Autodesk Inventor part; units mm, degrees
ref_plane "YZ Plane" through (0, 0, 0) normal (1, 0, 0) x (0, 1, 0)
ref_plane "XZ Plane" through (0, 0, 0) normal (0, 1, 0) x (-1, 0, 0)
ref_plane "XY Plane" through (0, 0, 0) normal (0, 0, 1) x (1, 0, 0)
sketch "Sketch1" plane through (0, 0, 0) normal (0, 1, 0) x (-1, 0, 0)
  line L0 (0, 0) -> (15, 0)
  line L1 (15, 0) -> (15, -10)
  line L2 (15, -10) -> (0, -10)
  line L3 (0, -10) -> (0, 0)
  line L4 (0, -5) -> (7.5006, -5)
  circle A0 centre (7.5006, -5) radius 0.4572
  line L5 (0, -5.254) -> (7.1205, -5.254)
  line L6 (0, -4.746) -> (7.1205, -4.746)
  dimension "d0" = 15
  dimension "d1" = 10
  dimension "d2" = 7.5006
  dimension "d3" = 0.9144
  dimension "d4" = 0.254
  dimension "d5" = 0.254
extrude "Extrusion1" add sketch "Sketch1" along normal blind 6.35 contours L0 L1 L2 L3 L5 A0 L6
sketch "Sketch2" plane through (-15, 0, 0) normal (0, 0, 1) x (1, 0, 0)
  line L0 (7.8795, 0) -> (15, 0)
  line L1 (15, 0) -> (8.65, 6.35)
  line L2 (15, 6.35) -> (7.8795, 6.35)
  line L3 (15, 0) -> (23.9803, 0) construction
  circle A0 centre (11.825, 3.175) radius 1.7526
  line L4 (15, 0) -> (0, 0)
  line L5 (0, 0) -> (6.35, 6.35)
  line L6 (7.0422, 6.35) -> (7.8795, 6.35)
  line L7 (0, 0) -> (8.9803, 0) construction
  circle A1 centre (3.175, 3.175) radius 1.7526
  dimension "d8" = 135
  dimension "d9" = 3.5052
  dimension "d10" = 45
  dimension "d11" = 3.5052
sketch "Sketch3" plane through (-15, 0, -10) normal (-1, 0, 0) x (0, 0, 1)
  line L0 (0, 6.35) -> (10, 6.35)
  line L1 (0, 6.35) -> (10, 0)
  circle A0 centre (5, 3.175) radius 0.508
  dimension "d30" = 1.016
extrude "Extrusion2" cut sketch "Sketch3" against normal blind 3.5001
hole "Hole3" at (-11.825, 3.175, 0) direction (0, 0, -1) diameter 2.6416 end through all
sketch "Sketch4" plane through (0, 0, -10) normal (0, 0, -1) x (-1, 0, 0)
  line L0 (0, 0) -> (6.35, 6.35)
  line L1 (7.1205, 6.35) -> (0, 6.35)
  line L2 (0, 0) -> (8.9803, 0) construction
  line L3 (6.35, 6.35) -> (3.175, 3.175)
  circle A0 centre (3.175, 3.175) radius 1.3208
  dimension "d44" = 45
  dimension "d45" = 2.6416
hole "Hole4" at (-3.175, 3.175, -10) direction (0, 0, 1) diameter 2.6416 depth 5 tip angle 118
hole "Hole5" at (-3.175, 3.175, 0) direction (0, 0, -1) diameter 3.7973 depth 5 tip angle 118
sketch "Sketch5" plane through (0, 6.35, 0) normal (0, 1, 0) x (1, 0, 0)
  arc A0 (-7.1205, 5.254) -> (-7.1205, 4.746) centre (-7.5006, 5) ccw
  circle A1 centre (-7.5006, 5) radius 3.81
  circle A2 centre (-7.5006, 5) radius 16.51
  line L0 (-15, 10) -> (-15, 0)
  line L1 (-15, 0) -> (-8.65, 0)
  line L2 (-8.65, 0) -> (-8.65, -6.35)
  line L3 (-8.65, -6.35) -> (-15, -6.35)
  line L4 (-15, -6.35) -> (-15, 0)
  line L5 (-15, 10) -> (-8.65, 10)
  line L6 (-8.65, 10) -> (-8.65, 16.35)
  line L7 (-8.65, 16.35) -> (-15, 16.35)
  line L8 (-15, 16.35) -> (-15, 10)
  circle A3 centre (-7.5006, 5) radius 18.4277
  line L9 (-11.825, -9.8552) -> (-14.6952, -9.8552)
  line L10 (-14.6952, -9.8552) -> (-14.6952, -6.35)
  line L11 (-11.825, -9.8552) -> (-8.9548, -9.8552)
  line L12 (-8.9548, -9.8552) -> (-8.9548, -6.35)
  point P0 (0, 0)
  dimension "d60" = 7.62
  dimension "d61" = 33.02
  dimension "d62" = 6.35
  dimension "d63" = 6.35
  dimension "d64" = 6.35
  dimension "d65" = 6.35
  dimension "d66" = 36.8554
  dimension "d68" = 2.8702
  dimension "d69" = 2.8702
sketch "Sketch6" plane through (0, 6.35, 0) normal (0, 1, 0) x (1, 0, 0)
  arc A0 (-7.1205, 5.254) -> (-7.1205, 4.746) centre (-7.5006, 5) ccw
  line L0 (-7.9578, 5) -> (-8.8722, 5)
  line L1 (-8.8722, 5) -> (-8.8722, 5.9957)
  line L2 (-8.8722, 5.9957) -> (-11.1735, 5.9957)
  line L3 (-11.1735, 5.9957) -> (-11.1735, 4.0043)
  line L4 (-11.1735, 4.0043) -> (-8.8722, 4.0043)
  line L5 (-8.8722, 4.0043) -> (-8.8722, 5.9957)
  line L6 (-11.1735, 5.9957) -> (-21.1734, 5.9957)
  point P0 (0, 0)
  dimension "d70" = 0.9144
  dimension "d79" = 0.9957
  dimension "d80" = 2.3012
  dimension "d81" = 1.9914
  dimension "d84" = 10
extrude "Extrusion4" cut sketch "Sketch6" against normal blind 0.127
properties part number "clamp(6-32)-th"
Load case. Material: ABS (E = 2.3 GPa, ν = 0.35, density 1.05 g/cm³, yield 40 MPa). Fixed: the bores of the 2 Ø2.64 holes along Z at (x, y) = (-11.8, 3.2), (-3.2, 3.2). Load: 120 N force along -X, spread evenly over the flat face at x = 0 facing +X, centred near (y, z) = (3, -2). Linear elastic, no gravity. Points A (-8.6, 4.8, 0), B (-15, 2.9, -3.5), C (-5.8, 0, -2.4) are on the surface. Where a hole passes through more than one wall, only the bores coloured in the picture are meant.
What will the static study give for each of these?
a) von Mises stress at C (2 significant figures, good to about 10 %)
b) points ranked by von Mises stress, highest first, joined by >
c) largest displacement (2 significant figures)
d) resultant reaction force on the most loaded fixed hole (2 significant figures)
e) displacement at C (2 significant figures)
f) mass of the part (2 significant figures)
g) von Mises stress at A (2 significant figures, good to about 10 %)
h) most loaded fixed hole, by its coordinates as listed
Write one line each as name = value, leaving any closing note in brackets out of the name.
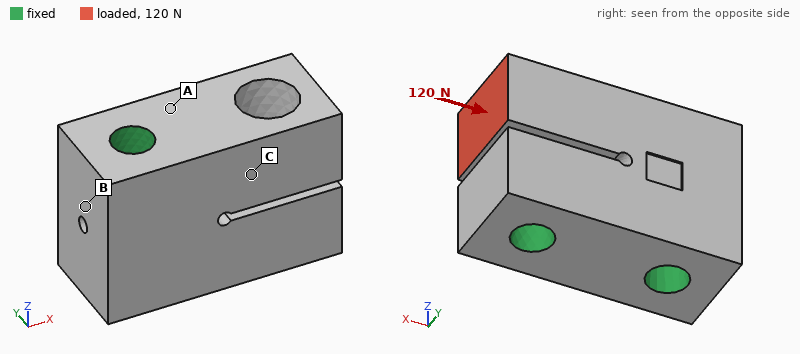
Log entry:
von Mises stress at C = 9.9 MPa
points ranked by von Mises stress, highest first, joined by > = C > A > B
largest displacement = 58 µm
resultant reaction force on the most loaded fixed hole = 120 N
displacement at C = 16 µm
mass of the part = 0.83 g
von Mises stress at A = 4.8 MPa
most loaded fixed hole, by its coordinates as listed = (-11.8, 3.2)
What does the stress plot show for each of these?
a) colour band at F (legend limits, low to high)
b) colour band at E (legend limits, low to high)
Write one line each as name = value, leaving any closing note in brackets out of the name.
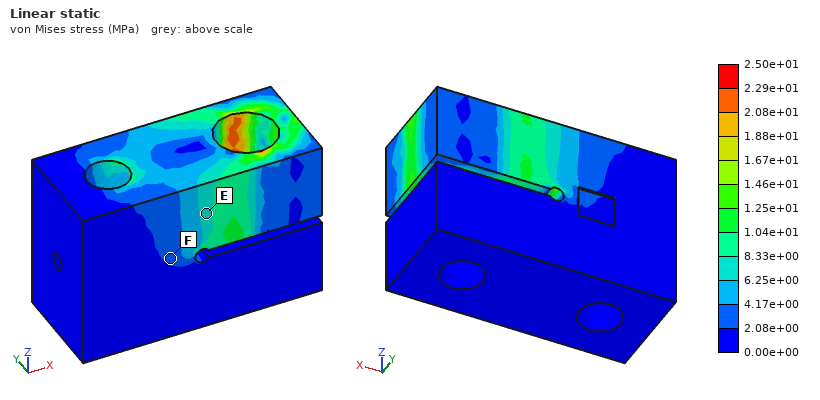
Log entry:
colour band at F = 2.08e+00 to 4.17e+00 MPa
colour band at E = 6.25e+00 to 8.33e+00 MPa
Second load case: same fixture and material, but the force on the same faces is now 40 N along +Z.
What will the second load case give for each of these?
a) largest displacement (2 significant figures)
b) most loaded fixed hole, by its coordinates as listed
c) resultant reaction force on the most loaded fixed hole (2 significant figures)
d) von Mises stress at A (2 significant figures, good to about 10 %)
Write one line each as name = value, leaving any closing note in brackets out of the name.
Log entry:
largest displacement = 0.17 mm
most loaded fixed hole, by its coordinates as listed = (-11.8, 3.2)
resultant reaction force on the most loaded fixed hole = 38 N
von Mises stress at A = 12 MPa
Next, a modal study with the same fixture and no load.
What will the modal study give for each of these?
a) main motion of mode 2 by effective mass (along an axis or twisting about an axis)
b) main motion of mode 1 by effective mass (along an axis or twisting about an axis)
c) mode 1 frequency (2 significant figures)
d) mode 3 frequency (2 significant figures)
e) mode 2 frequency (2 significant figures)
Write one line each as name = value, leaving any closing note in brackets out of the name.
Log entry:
main motion of mode 2 by effective mass = along Z
main motion of mode 1 by effective mass = along Y
mode 1 frequency = 9500 Hz
mode 3 frequency = 19 kHz
mode 2 frequency = 10 kHz
